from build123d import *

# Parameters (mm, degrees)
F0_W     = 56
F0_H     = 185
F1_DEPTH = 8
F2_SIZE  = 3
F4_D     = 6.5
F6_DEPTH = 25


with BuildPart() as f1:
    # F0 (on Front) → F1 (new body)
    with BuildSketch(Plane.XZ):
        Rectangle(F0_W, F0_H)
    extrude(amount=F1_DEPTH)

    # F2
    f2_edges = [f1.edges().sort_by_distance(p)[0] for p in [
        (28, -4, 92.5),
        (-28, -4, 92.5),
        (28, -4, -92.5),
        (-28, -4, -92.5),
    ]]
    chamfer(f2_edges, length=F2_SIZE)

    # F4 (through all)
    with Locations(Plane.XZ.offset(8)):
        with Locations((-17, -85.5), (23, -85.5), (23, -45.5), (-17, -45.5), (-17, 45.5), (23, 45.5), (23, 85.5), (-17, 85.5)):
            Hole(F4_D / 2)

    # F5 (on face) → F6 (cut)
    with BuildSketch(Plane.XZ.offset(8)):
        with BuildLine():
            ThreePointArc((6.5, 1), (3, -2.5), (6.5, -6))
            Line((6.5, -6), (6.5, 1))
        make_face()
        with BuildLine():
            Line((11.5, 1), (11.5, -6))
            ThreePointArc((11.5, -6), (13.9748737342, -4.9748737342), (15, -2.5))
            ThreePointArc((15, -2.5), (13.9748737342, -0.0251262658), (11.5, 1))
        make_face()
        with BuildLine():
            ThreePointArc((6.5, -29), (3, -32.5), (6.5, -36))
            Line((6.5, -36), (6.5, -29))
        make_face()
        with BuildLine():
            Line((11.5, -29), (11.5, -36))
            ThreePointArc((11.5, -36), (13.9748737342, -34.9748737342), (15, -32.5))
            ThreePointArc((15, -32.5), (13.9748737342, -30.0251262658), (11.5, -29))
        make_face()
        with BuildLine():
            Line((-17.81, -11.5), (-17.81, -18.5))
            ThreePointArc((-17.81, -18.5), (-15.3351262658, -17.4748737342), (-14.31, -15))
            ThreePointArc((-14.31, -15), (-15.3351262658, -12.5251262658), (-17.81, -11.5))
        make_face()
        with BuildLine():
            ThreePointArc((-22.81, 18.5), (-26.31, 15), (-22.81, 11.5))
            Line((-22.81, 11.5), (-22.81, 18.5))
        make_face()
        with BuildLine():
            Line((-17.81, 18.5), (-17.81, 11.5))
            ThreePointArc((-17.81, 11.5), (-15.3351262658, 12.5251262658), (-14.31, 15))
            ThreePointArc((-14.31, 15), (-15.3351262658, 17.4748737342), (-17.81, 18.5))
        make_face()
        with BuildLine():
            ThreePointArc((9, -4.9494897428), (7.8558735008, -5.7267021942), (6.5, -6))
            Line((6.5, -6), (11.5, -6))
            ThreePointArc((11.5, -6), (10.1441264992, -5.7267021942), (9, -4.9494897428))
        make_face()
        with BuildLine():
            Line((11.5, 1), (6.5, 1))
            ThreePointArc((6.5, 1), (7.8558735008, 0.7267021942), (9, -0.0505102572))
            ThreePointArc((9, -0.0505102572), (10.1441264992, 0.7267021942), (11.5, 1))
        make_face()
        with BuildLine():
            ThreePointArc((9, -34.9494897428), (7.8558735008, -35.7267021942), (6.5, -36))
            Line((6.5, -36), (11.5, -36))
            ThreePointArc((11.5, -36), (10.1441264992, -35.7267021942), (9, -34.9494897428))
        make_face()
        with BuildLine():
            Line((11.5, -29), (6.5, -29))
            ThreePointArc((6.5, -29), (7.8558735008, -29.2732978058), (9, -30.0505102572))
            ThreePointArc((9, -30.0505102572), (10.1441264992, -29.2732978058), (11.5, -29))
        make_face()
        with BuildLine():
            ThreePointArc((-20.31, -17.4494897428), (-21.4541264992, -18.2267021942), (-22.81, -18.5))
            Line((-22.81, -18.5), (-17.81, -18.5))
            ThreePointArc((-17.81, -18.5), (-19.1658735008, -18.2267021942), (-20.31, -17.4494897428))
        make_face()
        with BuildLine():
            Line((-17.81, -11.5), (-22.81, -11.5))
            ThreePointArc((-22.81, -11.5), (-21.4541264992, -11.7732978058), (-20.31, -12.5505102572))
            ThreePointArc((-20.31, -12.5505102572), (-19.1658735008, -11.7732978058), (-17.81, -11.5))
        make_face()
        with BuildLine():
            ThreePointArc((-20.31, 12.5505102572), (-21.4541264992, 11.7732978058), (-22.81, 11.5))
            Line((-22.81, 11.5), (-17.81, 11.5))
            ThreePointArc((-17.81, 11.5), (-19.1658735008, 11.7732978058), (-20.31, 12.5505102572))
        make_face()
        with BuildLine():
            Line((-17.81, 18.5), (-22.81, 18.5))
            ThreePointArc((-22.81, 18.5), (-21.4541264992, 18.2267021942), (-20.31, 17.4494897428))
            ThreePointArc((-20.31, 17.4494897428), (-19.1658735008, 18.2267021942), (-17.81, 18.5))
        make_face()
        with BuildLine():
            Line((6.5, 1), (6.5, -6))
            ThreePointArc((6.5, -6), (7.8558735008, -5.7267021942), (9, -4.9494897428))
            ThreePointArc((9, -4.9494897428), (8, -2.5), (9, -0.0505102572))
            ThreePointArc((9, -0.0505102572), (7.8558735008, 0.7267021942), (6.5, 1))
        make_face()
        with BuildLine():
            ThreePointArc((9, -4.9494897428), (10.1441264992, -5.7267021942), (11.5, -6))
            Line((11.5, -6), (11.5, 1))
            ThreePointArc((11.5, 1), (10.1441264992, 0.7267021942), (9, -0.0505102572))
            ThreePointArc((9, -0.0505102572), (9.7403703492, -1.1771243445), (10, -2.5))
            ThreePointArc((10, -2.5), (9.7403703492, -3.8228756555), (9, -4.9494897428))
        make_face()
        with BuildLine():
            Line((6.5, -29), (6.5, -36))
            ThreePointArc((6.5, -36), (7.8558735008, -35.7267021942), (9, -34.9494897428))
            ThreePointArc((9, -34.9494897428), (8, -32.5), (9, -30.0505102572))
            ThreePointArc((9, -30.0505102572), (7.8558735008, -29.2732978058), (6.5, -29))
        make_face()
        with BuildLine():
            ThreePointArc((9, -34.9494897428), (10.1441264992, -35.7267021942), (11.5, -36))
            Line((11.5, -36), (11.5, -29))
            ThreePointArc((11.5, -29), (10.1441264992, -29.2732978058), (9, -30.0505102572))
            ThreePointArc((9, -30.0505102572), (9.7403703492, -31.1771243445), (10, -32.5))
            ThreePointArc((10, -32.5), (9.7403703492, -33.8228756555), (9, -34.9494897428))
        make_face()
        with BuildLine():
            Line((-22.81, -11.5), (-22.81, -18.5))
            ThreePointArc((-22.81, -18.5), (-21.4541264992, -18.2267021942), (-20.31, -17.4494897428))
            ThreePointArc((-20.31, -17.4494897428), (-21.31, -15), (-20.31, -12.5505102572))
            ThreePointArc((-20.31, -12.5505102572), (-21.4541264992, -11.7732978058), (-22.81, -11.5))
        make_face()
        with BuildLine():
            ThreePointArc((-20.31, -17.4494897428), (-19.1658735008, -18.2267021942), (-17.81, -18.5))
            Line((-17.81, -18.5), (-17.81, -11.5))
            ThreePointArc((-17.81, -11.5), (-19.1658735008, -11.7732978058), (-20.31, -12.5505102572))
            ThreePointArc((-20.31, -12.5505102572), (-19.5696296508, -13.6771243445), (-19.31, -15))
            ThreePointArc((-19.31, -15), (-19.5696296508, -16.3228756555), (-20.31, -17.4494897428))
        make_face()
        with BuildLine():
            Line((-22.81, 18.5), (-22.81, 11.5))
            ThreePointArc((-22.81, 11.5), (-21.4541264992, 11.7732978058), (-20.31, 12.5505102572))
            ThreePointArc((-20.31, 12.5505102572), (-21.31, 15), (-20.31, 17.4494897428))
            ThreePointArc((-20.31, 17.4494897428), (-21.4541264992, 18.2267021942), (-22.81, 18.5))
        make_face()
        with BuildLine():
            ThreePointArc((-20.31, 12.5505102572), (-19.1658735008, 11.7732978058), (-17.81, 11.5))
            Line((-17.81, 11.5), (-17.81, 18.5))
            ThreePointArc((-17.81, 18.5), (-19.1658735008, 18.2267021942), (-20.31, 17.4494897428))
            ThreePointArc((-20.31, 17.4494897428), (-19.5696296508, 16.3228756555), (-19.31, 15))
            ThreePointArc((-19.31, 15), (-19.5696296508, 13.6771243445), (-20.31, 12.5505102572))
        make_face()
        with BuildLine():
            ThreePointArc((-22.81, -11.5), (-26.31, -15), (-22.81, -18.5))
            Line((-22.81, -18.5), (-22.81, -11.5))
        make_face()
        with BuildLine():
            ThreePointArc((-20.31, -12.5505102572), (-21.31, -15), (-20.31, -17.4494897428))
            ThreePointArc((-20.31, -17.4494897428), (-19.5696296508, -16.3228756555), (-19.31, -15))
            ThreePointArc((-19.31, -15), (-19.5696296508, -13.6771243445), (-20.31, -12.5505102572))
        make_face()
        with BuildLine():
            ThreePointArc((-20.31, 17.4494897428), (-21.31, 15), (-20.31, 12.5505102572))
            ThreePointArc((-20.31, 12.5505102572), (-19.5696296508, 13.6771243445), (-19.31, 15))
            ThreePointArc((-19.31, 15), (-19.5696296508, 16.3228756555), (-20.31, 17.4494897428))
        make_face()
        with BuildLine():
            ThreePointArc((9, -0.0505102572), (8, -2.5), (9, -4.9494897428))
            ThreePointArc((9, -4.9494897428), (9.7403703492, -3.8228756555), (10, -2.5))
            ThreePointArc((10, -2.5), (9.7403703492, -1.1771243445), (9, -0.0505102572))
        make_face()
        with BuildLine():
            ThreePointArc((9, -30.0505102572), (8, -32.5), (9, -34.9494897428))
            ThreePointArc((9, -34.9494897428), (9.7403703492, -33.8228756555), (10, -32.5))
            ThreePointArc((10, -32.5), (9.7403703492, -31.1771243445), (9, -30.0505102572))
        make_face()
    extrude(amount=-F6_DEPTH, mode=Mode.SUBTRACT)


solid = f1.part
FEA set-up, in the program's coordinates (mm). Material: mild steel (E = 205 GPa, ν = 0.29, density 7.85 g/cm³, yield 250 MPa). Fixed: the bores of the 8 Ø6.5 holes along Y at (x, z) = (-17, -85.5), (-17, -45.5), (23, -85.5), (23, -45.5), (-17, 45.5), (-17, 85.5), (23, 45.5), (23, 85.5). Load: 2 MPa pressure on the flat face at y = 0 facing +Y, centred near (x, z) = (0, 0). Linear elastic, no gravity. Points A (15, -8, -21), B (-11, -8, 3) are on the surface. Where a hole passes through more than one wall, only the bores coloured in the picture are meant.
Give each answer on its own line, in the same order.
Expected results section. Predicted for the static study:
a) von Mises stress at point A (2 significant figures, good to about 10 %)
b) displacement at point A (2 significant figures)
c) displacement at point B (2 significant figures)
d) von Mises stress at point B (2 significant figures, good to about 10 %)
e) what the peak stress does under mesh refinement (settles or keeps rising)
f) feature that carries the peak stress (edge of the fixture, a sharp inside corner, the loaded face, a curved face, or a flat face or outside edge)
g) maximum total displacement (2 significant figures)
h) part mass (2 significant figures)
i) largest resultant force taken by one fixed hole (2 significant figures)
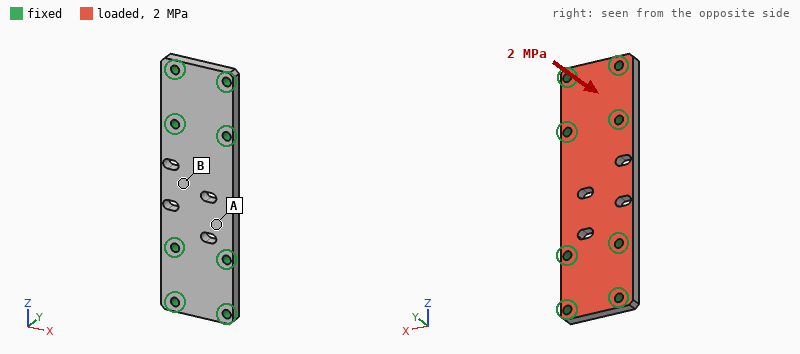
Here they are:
24 MPa
30 µm
45 µm
57 MPa
keeps rising
edge of the fixture
48 µm
610 g
4.1 kN
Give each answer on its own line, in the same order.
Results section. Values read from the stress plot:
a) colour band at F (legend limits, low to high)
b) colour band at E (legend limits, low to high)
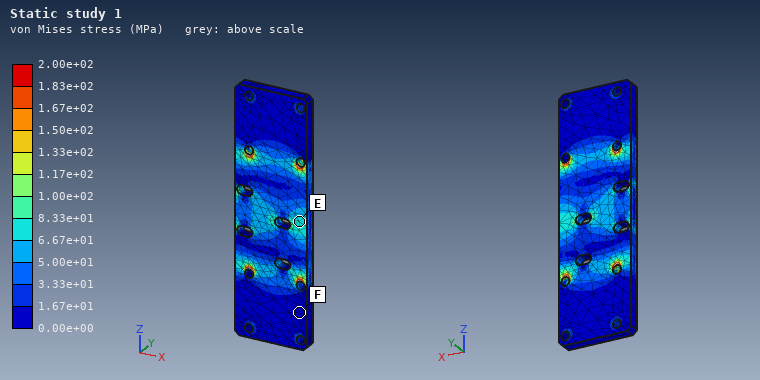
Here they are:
0.00e+00 to 1.67e+01 MPa
6.67e+01 to 8.33e+01 MPa
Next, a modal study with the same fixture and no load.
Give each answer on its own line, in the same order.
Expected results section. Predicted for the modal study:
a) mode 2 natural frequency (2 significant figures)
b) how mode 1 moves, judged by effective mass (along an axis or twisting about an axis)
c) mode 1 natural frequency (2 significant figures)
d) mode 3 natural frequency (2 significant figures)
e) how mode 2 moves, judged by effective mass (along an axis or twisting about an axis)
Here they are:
7000 Hz
along Y
4700 Hz
12 kHz
twisting about Z
